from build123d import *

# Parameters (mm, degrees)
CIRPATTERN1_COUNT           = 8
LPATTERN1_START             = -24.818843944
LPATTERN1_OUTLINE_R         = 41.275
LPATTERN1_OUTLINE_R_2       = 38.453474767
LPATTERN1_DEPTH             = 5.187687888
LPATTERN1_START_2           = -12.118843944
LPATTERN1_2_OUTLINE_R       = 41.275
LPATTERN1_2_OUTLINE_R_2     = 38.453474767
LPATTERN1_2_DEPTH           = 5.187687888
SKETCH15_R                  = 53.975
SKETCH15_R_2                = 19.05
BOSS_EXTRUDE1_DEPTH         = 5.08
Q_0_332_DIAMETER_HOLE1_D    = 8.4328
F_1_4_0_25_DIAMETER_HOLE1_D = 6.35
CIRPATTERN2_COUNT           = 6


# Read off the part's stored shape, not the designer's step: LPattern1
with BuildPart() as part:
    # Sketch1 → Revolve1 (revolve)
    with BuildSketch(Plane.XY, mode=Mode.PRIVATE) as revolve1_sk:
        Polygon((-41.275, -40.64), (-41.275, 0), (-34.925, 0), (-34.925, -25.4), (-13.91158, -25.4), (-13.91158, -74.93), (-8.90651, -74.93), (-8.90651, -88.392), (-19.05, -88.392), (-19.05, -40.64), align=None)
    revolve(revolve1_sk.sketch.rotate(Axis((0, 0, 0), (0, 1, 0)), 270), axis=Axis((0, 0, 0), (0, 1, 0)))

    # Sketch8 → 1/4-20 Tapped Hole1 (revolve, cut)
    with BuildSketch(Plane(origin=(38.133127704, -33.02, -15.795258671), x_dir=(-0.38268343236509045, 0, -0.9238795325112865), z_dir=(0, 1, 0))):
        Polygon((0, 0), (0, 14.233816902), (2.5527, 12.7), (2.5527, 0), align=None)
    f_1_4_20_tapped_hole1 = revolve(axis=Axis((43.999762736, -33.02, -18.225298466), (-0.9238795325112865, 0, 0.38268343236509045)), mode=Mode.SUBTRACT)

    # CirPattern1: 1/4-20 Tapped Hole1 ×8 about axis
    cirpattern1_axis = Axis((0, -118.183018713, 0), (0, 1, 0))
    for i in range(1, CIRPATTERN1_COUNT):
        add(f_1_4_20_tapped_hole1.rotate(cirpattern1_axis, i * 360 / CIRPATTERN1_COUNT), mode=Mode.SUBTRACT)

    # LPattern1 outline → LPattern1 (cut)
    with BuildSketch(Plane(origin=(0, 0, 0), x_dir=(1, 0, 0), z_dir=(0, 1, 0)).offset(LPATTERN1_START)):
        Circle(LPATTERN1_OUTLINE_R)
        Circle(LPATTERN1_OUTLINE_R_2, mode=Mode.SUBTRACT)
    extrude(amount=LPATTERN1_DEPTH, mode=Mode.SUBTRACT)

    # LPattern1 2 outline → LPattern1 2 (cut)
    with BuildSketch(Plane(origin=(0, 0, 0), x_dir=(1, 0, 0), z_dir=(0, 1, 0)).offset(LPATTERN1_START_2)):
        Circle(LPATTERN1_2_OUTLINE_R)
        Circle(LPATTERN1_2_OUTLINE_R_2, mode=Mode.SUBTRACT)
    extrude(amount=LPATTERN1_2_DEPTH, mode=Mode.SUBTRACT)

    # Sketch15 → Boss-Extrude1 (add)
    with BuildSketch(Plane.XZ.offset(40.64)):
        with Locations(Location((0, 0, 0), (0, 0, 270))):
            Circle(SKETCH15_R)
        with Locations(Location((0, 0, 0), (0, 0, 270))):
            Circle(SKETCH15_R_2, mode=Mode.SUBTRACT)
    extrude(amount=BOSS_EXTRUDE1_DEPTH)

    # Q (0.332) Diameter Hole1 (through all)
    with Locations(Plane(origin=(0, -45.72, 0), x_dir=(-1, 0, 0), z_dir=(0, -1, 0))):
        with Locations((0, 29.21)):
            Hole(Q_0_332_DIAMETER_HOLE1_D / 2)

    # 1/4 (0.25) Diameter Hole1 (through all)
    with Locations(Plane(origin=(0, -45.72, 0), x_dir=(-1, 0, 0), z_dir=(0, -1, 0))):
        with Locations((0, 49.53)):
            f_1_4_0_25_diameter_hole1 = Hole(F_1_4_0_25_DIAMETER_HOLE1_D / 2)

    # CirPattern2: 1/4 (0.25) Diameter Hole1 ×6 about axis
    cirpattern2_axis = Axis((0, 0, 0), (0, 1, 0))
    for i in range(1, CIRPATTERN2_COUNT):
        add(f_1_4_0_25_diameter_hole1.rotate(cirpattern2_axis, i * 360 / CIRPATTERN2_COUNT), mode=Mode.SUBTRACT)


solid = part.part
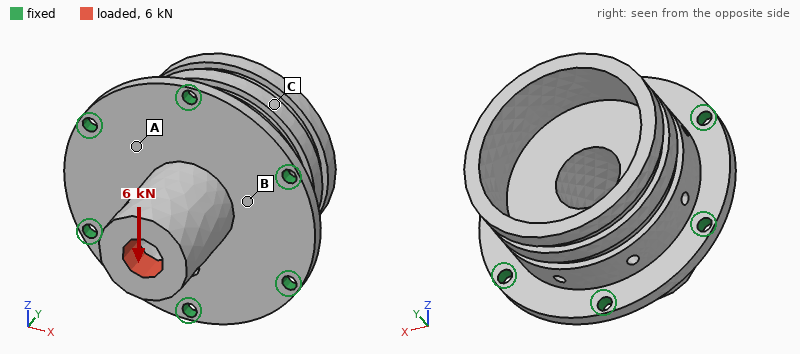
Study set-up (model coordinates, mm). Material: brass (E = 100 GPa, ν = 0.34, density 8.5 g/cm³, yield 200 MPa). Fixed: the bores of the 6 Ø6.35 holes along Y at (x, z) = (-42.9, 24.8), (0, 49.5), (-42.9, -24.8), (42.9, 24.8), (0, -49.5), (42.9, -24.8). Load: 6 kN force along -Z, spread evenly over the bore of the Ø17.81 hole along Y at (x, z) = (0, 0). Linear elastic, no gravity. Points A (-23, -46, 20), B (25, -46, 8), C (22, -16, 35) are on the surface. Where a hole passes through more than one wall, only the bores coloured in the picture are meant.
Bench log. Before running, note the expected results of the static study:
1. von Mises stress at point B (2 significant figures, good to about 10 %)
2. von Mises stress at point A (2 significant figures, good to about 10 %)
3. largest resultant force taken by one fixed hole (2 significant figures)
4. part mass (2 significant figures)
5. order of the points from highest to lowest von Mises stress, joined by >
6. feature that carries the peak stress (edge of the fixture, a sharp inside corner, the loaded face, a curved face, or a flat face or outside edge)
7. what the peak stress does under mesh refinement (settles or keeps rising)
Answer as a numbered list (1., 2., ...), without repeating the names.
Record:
1. 17 MPa
2. 9.1 MPa
3. 1.9 kN
4. 1.4 kg
5. B > A > C
6. edge of the fixture
7. keeps rising
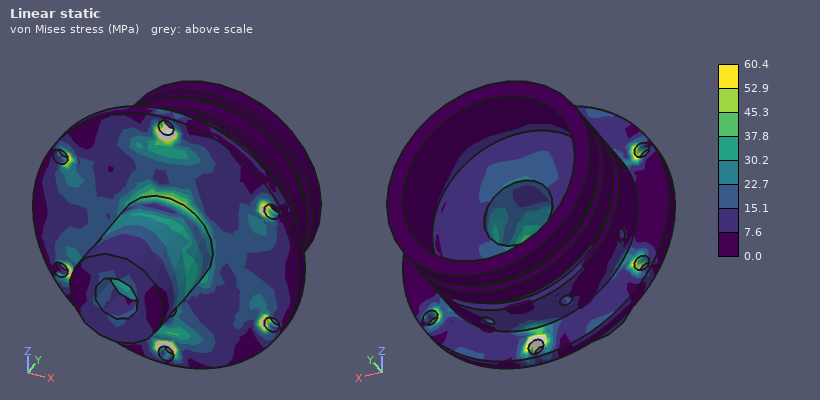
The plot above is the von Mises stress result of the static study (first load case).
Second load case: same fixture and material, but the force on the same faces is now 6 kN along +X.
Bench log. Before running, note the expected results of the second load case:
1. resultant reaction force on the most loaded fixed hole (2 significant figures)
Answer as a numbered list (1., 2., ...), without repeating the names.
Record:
1. 1.7 kN
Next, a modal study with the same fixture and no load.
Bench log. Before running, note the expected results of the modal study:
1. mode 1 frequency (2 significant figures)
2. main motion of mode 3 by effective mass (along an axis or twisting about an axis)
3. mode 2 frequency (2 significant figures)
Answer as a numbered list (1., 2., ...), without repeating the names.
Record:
1. 3600 Hz
2. along Y
3. 3600 Hz
